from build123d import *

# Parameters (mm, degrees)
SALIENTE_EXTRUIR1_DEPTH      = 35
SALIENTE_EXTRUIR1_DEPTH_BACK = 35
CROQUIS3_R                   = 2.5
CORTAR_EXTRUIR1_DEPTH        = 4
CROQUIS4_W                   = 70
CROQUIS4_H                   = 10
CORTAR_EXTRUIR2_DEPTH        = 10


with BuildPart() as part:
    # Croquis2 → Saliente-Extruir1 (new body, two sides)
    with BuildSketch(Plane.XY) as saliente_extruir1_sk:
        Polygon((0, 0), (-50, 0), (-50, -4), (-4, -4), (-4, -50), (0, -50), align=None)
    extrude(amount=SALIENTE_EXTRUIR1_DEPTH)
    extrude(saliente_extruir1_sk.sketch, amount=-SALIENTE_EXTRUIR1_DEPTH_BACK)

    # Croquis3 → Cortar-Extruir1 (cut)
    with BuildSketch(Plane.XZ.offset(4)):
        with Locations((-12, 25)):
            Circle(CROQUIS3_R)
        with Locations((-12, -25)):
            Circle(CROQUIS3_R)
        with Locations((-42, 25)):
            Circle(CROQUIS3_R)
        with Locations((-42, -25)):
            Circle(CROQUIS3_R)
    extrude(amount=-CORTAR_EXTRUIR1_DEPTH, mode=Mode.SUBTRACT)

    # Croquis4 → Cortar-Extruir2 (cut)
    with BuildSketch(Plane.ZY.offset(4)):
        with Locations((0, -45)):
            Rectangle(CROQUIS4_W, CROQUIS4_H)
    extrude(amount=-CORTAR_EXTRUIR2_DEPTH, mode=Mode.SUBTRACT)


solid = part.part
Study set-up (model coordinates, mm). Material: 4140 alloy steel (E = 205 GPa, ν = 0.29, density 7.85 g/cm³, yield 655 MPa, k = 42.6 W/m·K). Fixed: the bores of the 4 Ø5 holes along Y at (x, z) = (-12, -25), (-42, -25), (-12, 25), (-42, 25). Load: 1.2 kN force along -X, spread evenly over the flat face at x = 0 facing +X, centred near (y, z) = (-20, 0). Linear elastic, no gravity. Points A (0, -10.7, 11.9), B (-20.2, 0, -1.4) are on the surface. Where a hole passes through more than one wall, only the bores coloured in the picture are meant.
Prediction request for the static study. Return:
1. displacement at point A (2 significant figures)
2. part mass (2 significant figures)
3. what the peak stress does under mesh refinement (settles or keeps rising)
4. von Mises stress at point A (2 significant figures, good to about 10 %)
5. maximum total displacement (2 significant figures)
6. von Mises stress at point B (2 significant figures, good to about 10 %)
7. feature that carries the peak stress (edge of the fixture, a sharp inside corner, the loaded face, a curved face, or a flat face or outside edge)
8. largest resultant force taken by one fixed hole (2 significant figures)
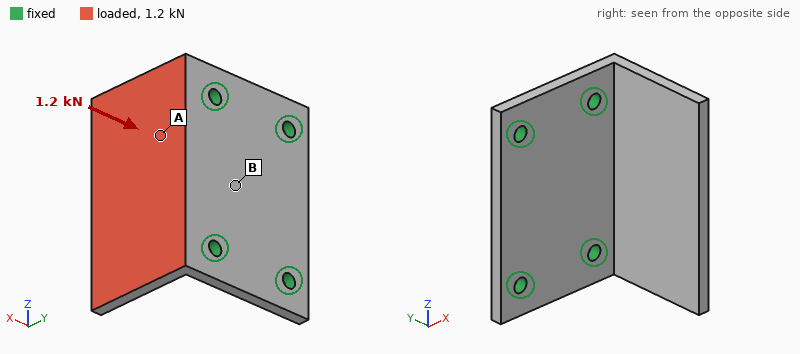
0.040 mm
190 g
keeps rising
61 MPa
0.20 mm
27 MPa
edge of the fixture
460 N
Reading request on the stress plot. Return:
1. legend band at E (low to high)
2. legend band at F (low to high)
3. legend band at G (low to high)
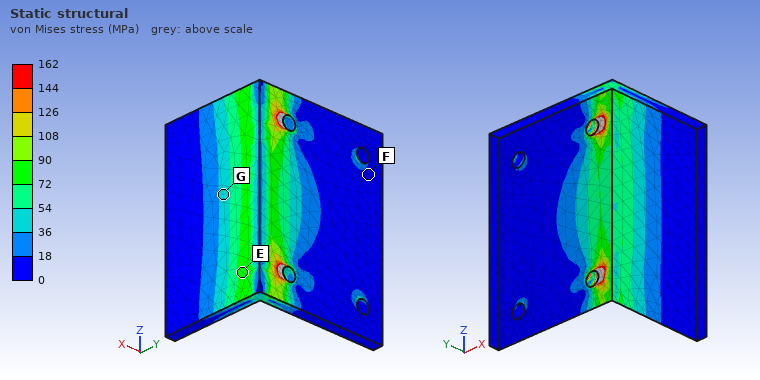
72 to 90 MPa
0 to 18 MPa
36 to 54 MPa
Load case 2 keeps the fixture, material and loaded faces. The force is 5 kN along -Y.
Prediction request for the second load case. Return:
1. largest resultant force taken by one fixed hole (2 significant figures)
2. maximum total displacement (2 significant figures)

2.8 kN
0.25 mm
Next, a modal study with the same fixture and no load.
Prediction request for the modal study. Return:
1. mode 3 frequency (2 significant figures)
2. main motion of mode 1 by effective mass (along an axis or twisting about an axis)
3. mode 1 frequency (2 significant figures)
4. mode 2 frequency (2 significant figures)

6800 Hz
along X
1600 Hz
3100 Hz
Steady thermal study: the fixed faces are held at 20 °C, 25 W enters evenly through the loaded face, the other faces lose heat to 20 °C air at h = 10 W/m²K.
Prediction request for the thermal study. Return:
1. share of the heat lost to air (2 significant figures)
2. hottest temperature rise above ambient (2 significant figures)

8.5 %
61 K
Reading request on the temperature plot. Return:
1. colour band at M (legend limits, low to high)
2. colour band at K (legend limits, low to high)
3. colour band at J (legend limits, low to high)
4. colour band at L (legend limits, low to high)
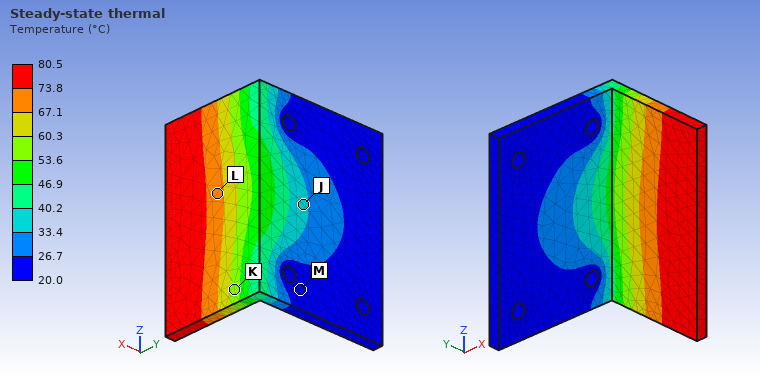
20.0 to 26.7 °C
53.6 to 60.3 °C
33.4 to 40.2 °C
67.1 to 73.8 °C
